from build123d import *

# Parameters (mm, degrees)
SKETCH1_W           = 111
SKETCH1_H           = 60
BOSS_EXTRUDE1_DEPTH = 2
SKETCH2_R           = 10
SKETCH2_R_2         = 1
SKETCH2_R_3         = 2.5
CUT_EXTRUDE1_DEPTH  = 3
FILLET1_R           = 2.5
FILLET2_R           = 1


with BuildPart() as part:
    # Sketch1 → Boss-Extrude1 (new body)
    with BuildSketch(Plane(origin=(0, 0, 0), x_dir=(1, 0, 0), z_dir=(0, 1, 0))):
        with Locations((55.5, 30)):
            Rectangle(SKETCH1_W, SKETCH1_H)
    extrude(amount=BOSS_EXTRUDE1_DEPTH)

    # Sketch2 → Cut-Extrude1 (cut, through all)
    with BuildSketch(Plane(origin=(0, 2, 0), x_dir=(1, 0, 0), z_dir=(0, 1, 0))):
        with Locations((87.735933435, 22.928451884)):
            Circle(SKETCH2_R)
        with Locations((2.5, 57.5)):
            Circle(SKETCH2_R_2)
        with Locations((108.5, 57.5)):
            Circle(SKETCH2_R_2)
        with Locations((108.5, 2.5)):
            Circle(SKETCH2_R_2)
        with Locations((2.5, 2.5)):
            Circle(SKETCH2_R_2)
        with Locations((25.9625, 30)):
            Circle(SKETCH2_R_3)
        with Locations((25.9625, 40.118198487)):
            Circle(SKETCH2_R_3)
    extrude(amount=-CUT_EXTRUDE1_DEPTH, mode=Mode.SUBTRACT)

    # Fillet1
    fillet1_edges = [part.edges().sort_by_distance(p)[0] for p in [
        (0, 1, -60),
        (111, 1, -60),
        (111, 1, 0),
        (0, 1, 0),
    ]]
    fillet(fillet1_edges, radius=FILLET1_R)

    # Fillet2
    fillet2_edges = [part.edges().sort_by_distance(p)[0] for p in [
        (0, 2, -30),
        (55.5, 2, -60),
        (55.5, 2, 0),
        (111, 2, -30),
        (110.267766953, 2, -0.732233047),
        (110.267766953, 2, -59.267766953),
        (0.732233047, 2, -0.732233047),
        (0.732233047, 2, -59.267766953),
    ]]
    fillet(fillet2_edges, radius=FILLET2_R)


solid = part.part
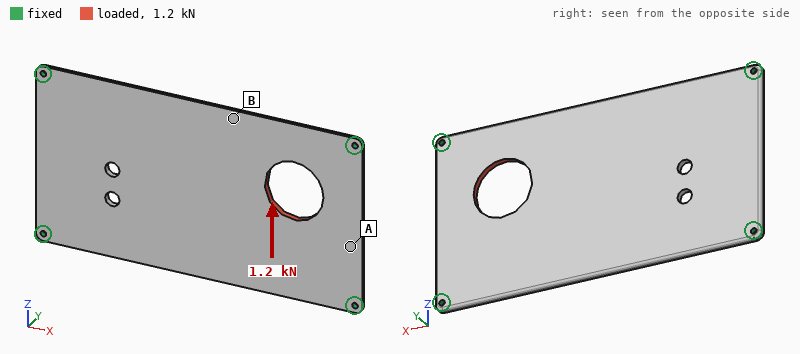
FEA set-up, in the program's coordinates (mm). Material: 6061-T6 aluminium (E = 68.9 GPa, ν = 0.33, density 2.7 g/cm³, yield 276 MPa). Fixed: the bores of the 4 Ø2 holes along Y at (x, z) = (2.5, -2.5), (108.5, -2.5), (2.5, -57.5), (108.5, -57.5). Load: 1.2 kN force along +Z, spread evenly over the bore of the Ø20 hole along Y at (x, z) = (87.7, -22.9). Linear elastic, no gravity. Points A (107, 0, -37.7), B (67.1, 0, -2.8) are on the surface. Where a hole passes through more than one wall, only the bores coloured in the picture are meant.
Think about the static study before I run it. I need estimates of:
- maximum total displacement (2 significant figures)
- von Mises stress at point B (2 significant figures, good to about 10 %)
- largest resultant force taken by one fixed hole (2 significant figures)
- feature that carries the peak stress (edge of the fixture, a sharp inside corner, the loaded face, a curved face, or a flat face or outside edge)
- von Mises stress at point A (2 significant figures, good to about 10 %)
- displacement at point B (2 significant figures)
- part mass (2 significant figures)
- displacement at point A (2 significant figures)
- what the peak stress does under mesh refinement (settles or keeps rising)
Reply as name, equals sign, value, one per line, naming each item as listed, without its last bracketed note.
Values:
maximum total displacement = 18 µm
von Mises stress at point B = 4.8 MPa
largest resultant force taken by one fixed hole = 510 N
feature that carries the peak stress = edge of the fixture
von Mises stress at point A = 11 MPa
displacement at point B = 14 µm
part mass = 34 g
displacement at point A = 6.7 µm
what the peak stress does under mesh refinement = keeps rising
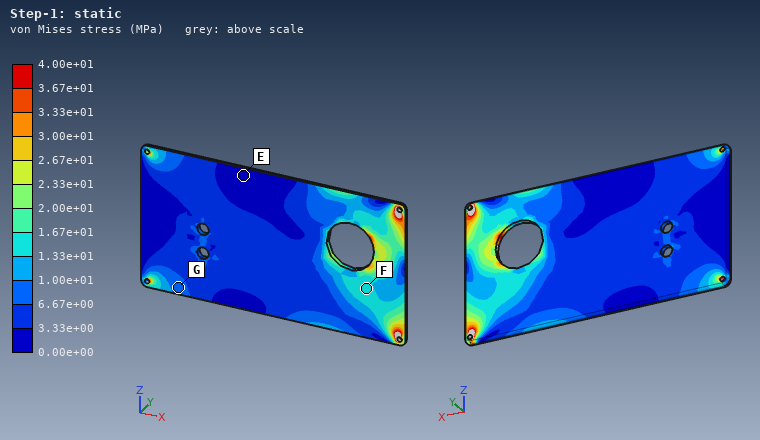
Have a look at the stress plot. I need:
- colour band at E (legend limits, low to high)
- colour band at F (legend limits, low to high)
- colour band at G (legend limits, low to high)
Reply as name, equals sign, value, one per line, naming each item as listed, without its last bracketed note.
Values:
colour band at E = 0.00e+00 to 3.33e+00 MPa
colour band at F = 1.33e+01 to 1.67e+01 MPa
colour band at G = 6.67e+00 to 1.00e+01 MPa
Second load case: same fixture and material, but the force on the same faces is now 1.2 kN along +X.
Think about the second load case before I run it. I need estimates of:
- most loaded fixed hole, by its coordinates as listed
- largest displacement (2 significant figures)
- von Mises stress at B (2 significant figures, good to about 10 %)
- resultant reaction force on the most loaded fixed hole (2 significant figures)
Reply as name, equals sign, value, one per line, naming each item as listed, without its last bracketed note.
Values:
most loaded fixed hole, by its coordinates as listed = (108.5, -2.5)
largest displacement = 13 µm
von Mises stress at B = 4.1 MPa
resultant reaction force on the most loaded fixed hole = 470 N
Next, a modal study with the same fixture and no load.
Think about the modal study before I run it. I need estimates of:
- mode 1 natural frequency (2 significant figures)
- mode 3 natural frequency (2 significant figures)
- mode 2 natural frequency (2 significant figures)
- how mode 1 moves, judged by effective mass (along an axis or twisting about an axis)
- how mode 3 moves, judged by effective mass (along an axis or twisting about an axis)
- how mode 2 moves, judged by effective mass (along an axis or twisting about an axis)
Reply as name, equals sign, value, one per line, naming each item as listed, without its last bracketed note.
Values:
mode 1 natural frequency = 710 Hz
mode 3 natural frequency = 2000 Hz
mode 2 natural frequency = 1300 Hz
how mode 1 moves, judged by effective mass = along Y
how mode 3 moves, judged by effective mass = twisting about Z
how mode 2 moves, judged by effective mass = twisting about X
